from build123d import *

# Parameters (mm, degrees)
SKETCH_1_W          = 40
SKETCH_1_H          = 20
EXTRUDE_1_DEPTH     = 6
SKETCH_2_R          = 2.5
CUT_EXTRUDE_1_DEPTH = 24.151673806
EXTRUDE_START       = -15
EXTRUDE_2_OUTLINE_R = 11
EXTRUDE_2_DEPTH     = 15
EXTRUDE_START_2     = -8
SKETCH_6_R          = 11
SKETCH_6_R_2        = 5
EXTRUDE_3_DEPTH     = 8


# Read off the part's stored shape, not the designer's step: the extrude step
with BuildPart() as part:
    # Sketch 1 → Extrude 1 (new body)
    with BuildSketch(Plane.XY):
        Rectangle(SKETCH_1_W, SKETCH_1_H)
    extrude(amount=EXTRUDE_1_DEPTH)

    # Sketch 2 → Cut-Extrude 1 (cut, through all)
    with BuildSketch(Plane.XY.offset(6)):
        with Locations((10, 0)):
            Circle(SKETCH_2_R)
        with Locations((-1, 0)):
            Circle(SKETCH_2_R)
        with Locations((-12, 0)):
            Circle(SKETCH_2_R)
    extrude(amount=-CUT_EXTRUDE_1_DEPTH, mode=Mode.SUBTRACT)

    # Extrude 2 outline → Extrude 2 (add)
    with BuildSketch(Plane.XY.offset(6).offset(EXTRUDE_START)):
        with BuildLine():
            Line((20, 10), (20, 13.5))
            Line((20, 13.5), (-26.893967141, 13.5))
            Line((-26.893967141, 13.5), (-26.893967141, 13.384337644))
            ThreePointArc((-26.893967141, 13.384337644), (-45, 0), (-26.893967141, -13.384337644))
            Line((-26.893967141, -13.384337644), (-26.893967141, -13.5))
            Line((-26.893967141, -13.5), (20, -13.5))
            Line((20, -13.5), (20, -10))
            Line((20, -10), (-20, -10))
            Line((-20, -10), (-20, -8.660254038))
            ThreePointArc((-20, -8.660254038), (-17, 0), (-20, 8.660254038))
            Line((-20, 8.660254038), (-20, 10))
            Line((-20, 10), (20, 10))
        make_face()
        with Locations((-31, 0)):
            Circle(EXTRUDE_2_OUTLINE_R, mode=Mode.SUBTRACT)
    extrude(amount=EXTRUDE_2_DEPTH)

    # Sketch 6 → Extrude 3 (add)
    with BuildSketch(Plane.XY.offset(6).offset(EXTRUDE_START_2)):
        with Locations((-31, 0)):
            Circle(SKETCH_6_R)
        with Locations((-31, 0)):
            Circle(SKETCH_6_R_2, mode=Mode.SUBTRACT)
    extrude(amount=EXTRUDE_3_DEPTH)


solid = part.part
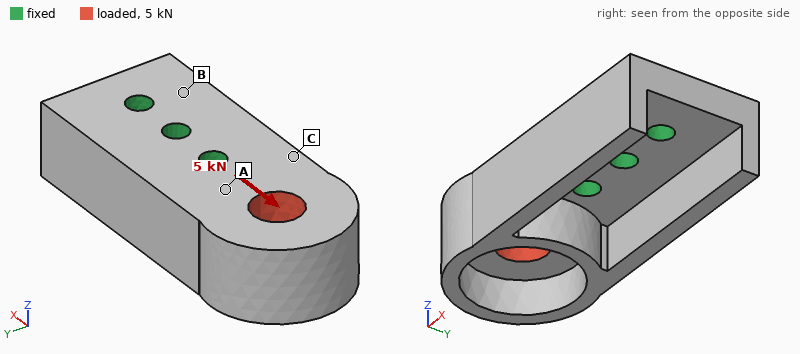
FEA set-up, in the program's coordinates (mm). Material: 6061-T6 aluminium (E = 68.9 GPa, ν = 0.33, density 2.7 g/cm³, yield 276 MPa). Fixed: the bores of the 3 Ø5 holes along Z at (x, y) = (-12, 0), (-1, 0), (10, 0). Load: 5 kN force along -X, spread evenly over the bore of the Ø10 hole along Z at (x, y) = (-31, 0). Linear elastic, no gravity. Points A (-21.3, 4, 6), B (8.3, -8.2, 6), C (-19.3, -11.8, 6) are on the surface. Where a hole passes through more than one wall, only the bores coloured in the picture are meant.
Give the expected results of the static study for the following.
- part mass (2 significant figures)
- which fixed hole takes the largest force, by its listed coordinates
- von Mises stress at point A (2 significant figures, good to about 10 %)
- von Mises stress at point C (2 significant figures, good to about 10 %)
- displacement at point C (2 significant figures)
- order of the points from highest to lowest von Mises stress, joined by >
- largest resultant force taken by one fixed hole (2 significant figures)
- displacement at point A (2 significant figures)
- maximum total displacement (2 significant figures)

40 g
(-12, 0)
40 MPa
20 MPa
6.3 µm
A > C > B
3.4 kN
4.9 µm
16 µm
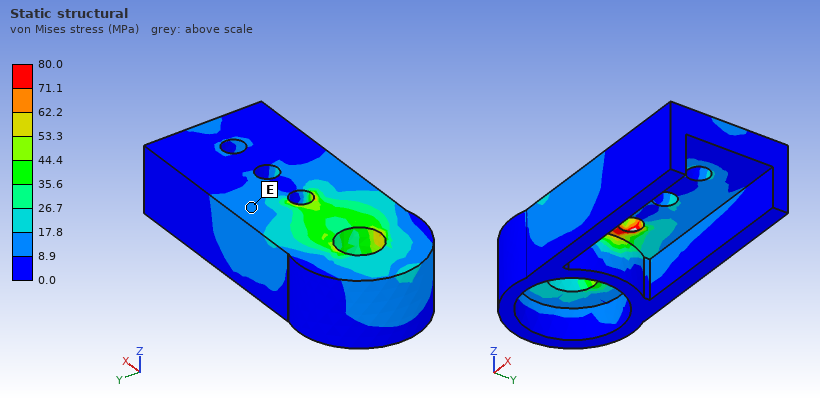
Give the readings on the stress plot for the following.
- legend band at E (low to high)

8.9 to 17.8 MPa
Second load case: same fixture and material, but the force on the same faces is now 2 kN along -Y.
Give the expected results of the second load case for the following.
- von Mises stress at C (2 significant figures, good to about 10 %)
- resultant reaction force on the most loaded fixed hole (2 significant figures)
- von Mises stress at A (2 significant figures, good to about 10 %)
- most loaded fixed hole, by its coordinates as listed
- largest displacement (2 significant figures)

22 MPa
3.4 kN
19 MPa
(-12, 0)
43 µm
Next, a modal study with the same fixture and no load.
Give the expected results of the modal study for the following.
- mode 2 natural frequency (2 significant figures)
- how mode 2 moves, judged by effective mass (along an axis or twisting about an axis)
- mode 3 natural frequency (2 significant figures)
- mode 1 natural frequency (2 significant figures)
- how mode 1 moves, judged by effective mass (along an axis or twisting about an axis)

8300 Hz
along Y
10 kHz
6300 Hz
along Z
